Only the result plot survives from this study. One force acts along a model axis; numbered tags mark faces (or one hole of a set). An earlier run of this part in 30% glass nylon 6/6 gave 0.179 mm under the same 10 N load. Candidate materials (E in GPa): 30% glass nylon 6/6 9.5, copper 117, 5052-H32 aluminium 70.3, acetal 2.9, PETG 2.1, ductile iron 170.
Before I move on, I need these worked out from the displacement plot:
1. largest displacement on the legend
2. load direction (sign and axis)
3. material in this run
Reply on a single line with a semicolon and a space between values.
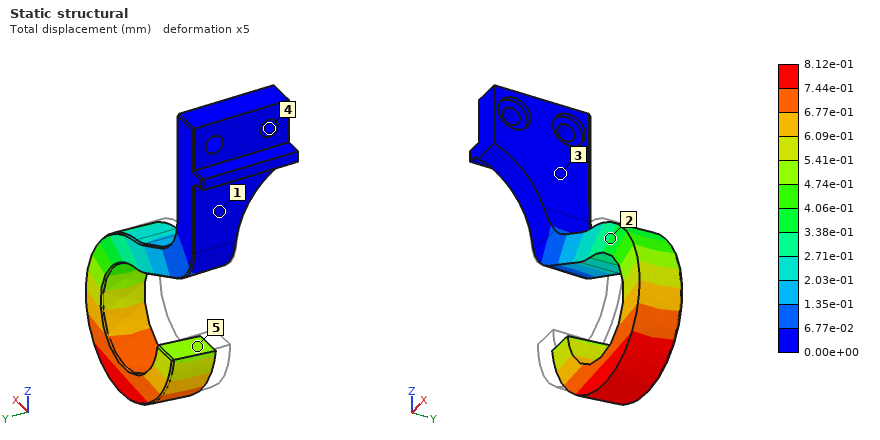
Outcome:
8.12e-01 mm; +Y; PETG
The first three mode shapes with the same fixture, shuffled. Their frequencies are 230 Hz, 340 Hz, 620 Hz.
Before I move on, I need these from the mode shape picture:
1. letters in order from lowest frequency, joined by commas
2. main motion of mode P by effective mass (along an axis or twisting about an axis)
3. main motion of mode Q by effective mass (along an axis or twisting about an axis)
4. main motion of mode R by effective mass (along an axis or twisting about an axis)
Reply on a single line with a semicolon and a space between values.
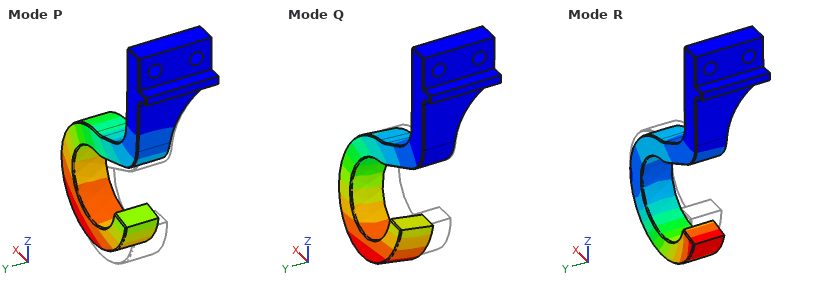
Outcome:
P, Q, R; along X; along Y; along Z
